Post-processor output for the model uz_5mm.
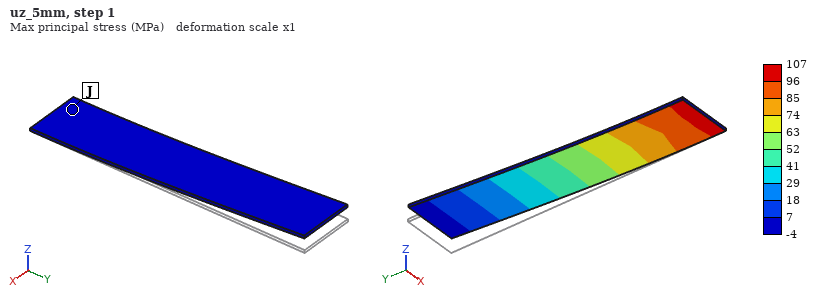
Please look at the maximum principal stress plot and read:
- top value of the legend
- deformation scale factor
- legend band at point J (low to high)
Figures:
107 MPa
1
-4 to 7 MPa
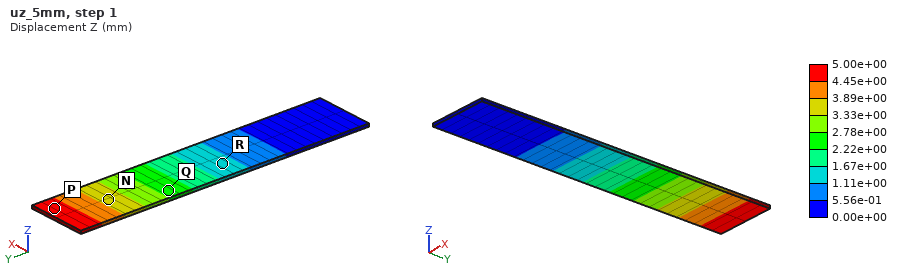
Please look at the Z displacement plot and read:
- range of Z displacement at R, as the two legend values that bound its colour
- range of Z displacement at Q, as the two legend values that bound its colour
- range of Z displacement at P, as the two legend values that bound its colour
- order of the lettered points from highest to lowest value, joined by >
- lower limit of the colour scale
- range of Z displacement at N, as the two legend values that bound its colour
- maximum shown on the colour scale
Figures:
1.11e+00 to 1.67e+00 mm
2.22e+00 to 2.78e+00 mm
4.45e+00 to 5.00e+00 mm
P > N > Q > R
0.00e+00 mm
3.33e+00 to 3.89e+00 mm
5.00e+00 mm
